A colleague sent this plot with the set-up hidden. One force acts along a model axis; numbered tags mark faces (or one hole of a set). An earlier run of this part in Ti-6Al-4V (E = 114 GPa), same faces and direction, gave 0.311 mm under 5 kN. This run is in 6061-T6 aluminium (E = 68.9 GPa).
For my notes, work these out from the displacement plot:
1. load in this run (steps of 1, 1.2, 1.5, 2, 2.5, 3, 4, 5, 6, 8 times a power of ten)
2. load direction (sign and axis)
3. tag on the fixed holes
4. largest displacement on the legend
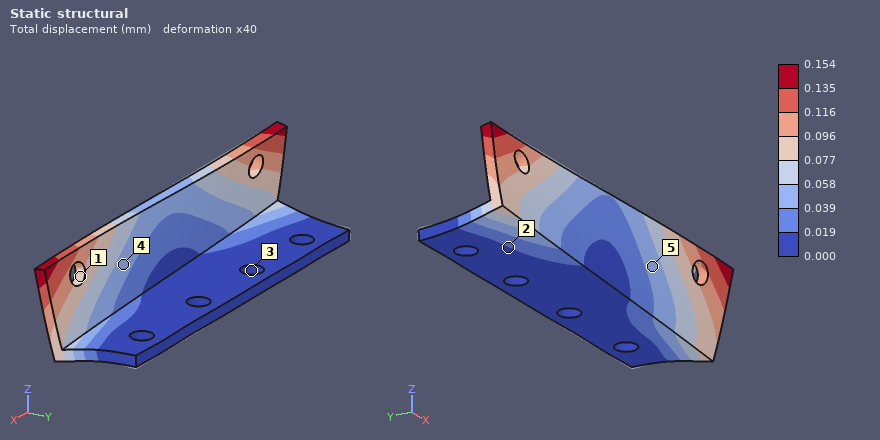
1.5 kN
+X
3
0.154 mm
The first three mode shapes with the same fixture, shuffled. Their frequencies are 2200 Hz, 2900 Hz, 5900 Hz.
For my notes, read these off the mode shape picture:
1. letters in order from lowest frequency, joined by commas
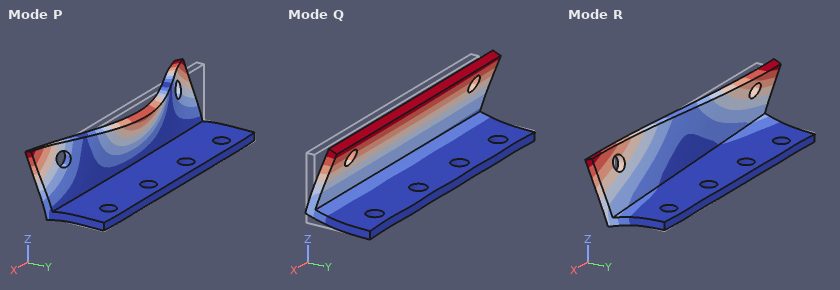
Q, R, P
